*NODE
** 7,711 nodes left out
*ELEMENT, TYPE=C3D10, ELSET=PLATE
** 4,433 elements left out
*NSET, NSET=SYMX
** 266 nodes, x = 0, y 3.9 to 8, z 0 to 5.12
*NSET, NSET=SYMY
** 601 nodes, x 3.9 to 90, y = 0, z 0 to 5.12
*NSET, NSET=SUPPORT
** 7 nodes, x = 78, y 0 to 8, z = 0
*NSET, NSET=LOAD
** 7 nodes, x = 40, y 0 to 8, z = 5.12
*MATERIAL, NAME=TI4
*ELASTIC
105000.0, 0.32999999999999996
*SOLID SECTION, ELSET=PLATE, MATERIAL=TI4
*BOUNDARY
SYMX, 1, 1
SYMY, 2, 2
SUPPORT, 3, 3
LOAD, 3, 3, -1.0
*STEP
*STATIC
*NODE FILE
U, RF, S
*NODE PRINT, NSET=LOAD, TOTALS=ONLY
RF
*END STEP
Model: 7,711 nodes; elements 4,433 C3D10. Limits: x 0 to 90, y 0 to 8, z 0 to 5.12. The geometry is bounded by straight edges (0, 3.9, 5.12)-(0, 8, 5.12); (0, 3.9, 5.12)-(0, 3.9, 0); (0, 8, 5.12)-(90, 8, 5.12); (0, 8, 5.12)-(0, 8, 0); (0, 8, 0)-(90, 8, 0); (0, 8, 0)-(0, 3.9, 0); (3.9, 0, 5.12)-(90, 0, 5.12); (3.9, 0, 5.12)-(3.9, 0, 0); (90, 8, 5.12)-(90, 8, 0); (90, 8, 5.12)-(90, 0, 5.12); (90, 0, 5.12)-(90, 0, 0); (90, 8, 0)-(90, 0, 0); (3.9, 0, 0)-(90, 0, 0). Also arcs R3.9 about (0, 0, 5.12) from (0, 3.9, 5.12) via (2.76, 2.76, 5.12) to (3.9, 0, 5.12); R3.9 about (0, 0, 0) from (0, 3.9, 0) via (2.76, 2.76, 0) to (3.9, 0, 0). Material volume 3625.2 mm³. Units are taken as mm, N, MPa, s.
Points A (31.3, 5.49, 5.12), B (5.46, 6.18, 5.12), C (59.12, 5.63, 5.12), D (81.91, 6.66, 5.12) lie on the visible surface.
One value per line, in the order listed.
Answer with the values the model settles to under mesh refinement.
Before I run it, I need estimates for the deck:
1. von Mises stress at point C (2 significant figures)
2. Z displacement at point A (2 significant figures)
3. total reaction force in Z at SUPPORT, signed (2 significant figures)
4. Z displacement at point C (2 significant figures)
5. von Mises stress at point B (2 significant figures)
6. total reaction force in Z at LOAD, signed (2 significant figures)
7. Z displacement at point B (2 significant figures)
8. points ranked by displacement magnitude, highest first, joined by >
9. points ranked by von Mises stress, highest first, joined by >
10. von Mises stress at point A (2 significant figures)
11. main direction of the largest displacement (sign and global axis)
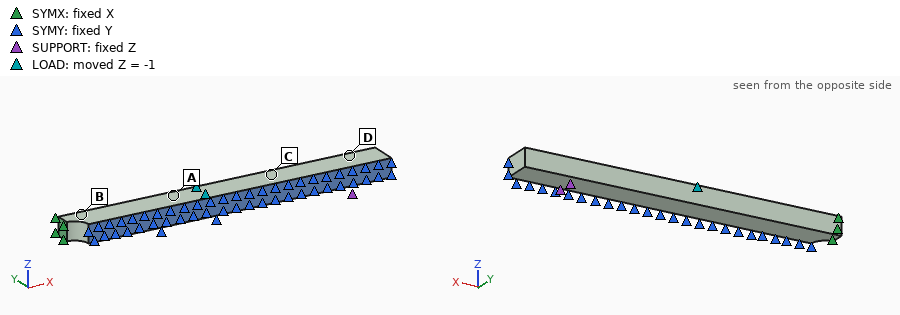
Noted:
62 MPa
-1.2 mm
110 N
-0.54 mm
170 MPa
-110 N
-1.4 mm
B > A > C > D
B > A > C > D
120 MPa
-Z
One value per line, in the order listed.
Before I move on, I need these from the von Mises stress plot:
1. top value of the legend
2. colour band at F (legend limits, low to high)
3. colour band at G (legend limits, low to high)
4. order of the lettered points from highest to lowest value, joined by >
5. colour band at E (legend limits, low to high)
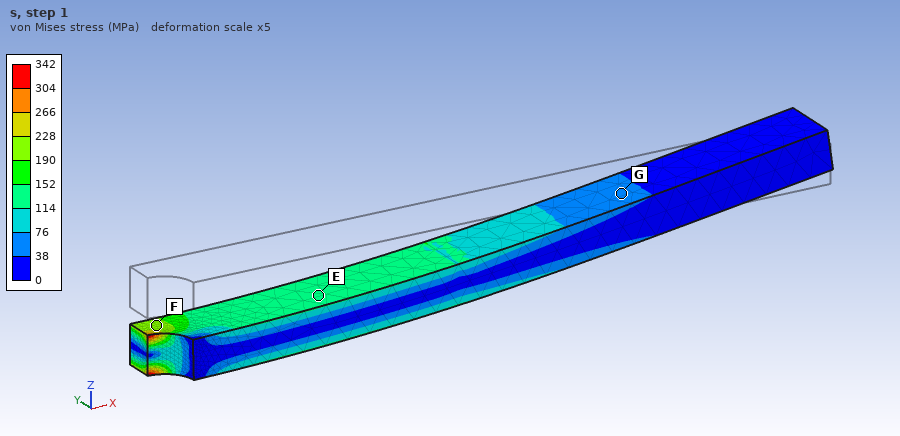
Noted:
342 MPa
190 to 228 MPa
38 to 76 MPa
F > E > G
114 to 152 MPa
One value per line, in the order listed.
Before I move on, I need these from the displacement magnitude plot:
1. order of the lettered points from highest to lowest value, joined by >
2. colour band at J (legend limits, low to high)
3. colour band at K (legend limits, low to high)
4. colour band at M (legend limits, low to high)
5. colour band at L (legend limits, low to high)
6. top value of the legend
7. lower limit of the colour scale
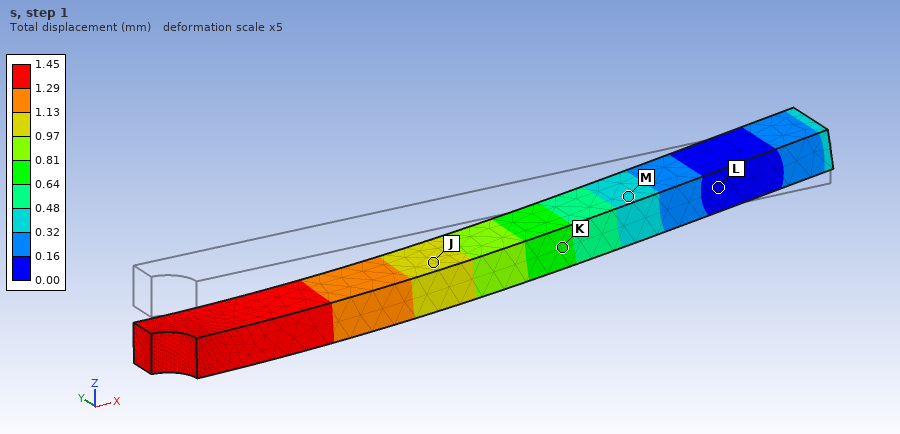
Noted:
J > K > M > L
0.97 to 1.13 mm
0.64 to 0.81 mm
0.32 to 0.48 mm
0.00 to 0.16 mm
1.45 mm
0.00 mm
